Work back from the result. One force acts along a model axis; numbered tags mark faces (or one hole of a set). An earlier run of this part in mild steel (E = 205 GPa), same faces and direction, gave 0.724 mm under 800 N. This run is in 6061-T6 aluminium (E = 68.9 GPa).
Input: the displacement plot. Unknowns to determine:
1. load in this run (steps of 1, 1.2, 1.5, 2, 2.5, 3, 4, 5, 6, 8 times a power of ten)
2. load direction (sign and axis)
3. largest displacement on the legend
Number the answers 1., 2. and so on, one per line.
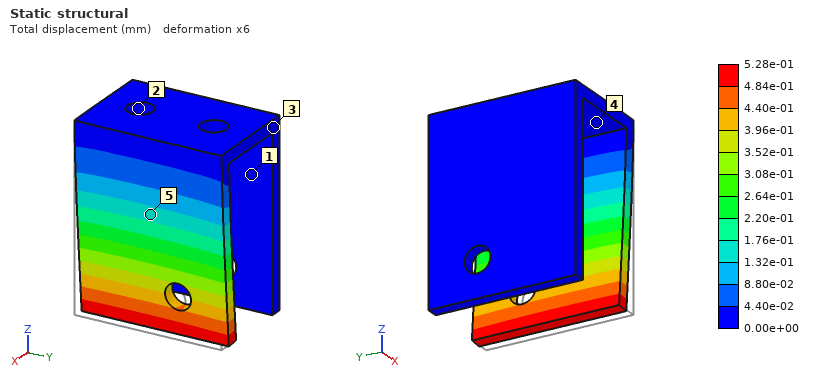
1. 200 N
2. -X
3. 5.28e-01 mm
